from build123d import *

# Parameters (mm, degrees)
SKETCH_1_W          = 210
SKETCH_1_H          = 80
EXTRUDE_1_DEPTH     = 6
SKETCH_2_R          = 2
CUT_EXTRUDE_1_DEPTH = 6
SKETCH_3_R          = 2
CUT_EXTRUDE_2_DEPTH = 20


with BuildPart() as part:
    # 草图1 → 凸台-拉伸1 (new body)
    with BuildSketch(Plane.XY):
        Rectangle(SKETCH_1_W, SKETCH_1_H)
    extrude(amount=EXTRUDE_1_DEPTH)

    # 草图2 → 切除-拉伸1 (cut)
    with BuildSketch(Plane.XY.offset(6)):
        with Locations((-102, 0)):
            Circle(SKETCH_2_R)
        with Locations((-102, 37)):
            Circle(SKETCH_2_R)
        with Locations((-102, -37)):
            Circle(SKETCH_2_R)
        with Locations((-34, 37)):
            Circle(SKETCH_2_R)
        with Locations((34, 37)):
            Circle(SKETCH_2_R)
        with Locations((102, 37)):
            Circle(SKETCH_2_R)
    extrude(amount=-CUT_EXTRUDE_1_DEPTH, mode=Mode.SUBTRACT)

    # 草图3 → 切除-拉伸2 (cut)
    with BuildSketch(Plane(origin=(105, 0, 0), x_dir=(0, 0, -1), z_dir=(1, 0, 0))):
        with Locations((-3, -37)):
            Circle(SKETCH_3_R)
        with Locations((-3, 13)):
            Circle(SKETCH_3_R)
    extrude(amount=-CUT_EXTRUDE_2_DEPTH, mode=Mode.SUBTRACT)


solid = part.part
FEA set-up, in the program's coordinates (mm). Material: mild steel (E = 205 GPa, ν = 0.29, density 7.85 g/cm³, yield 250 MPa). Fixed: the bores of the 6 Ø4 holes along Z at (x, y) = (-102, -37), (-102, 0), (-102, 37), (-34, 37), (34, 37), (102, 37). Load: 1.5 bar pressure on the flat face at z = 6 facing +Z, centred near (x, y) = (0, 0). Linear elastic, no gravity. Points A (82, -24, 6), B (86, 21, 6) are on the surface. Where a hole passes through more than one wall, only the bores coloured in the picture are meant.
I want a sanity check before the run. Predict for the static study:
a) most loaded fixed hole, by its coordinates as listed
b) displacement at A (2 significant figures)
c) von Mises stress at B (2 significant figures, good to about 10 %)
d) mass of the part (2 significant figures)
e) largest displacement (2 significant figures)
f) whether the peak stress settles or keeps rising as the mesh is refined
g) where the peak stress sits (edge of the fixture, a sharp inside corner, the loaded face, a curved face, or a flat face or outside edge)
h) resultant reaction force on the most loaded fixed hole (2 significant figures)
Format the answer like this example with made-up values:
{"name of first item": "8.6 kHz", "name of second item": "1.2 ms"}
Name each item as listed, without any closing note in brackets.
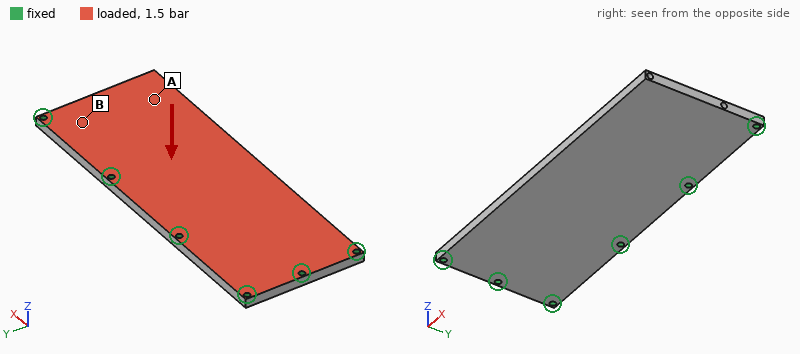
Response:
{"most loaded fixed hole, by its coordinates as listed": "(34, 37)", "displacement at A": "0.22 mm", "von Mises stress at B": "40 MPa", "mass of the part": "780 g", "largest displacement": "0.28 mm", "whether the peak stress settles or keeps rising as the mesh is refined": "keeps rising", "where the peak stress sits": "edge of the fixture", "resultant reaction force on the most loaded fixed hole": "900 N"}
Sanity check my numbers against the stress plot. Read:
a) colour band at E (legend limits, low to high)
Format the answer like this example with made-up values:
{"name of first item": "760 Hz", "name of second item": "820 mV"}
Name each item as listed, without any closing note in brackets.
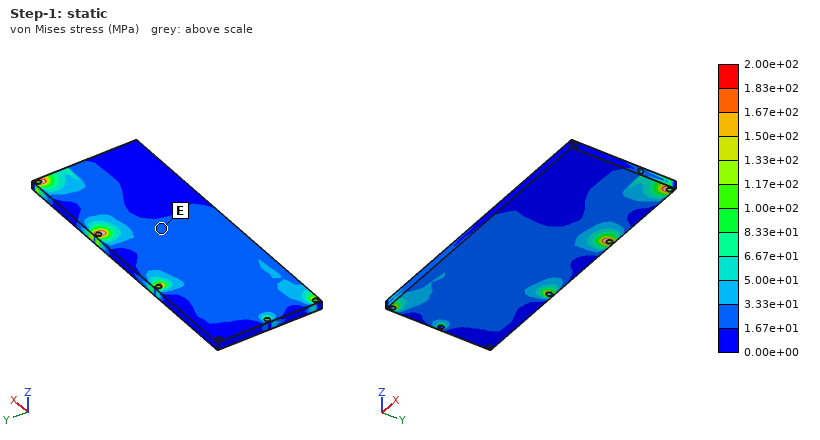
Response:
{"colour band at E": "1.67e+01 to 3.33e+01 MPa"}
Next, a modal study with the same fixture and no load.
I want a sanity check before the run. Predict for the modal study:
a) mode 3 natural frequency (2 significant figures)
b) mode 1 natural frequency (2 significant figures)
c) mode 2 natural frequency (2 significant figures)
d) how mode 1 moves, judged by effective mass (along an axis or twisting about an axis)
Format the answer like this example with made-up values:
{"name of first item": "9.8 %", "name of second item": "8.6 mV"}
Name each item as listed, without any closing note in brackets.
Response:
{"mode 3 natural frequency": "2700 Hz", "mode 1 natural frequency": "720 Hz", "mode 2 natural frequency": "1400 Hz", "how mode 1 moves, judged by effective mass": "along Z"}
